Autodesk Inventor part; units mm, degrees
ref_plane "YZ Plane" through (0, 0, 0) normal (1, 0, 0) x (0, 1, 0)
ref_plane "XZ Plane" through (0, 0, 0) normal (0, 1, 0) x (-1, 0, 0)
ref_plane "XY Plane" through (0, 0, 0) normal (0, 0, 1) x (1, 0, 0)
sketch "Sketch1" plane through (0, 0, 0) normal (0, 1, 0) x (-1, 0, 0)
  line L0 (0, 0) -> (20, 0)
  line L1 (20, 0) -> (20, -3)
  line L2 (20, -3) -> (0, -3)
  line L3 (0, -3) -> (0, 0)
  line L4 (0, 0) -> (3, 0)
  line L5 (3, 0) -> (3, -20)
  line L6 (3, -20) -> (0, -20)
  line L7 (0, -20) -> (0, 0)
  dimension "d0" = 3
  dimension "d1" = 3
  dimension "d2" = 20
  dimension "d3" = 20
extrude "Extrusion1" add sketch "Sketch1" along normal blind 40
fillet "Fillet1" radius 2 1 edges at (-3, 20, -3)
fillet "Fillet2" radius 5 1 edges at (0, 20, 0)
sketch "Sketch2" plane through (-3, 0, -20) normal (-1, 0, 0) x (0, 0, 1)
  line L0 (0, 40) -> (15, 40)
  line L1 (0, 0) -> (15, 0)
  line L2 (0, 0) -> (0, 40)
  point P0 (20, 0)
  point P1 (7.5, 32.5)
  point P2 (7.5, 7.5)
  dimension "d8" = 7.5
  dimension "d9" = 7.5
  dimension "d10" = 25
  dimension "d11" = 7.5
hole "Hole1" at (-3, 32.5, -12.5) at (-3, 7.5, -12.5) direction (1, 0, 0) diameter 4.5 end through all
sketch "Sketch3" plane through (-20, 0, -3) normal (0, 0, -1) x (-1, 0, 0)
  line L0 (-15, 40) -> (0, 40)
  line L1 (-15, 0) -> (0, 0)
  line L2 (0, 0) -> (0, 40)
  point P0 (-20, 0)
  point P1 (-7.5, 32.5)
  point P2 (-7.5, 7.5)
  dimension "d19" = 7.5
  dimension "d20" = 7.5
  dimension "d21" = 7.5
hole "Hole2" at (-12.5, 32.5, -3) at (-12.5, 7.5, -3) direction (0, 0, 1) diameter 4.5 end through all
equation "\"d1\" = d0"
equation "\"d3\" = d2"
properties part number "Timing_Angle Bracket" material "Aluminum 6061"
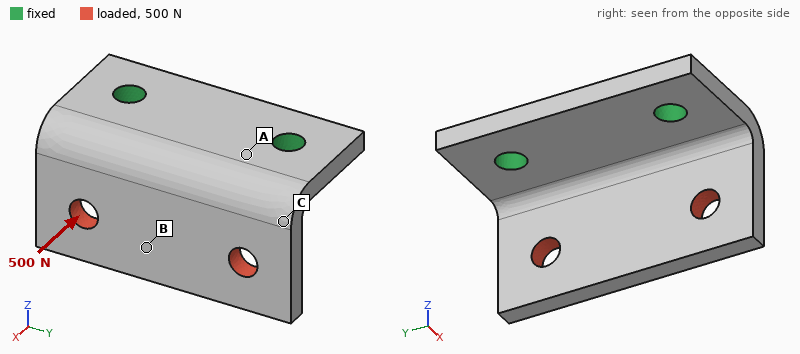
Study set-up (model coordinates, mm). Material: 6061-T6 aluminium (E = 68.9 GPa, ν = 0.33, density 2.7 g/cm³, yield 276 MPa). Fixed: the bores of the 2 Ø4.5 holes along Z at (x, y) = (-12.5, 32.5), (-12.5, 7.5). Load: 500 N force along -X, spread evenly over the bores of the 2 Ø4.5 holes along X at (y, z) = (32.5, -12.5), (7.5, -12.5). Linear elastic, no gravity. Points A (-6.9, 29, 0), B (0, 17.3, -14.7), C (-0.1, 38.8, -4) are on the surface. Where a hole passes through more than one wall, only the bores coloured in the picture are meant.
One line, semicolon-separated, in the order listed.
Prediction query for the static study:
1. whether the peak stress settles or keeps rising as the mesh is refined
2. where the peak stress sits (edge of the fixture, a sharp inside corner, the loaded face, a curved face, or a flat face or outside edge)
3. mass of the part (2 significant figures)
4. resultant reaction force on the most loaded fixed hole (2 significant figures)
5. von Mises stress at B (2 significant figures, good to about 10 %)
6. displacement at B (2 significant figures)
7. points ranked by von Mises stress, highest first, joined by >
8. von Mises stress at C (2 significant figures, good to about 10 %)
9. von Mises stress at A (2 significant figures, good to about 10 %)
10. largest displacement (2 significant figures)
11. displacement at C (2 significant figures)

keeps rising; edge of the fixture; 11 g; 250 N; 15 MPa; 0.15 mm; A > C > B; 53 MPa; 80 MPa; 0.22 mm; 0.065 mm
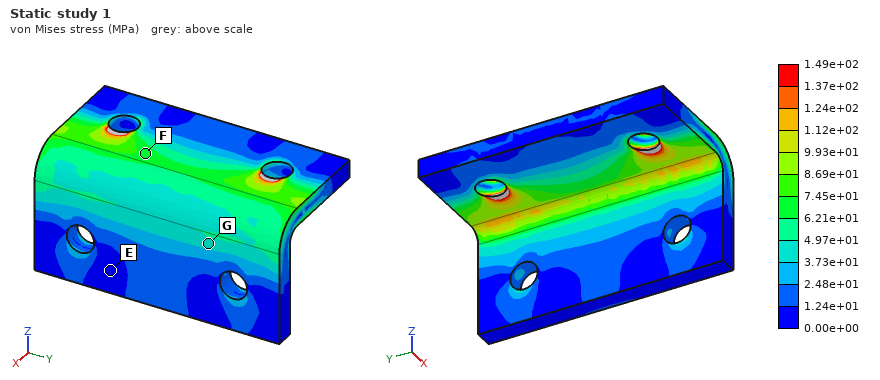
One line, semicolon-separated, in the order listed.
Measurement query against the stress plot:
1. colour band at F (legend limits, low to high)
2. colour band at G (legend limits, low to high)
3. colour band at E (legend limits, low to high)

6.21e+01 to 7.45e+01 MPa; 3.73e+01 to 4.97e+01 MPa; 0.00e+00 to 1.24e+01 MPa
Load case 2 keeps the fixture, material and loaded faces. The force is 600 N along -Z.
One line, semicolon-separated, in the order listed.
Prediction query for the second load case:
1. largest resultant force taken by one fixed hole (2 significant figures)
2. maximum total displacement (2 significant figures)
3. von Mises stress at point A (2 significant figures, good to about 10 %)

300 N; 0.11 mm; 52 MPa
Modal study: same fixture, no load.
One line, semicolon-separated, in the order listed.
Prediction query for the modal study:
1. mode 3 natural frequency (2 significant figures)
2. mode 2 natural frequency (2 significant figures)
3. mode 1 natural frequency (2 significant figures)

12 kHz; 6800 Hz; 4000 Hz
